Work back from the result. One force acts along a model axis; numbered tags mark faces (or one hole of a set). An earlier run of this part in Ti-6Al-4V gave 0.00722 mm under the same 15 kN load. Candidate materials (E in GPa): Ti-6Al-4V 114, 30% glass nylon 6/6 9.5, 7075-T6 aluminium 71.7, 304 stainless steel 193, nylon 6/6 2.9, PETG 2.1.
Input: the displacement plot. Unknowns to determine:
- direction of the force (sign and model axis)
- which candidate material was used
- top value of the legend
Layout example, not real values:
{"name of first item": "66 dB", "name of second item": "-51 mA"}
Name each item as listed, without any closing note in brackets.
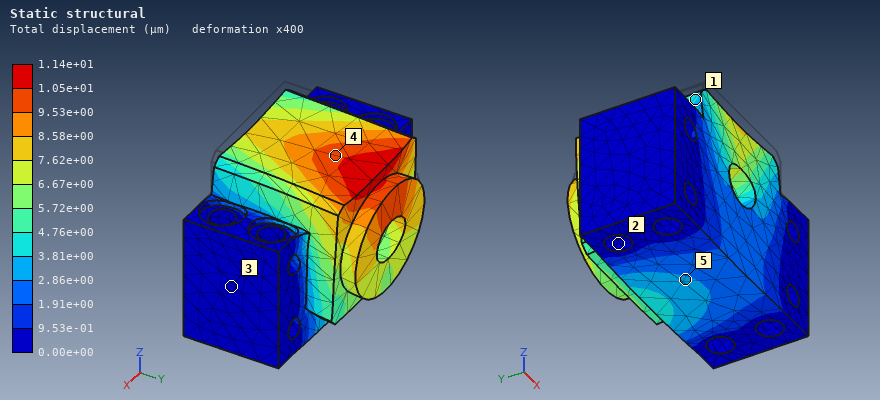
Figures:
{"direction of the force": "-Z", "which candidate material was used": "7075-T6 aluminium", "top value of the legend": "1.14e+01 µm"}
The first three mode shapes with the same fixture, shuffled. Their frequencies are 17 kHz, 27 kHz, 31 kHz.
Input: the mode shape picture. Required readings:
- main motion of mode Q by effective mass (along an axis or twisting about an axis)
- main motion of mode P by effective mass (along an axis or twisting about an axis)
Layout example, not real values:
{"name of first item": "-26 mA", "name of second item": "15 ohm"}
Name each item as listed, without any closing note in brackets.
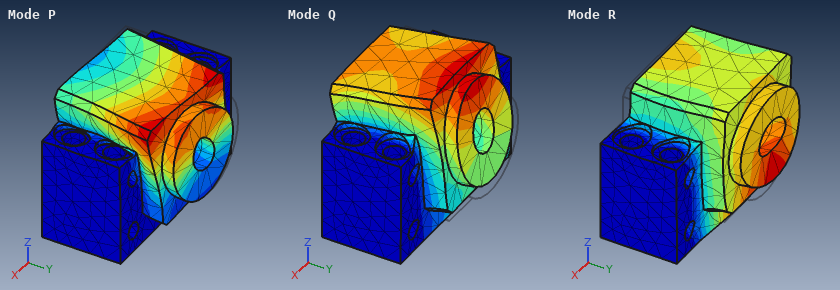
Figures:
{"main motion of mode Q by effective mass": "along Y", "main motion of mode P by effective mass": "along X"}
